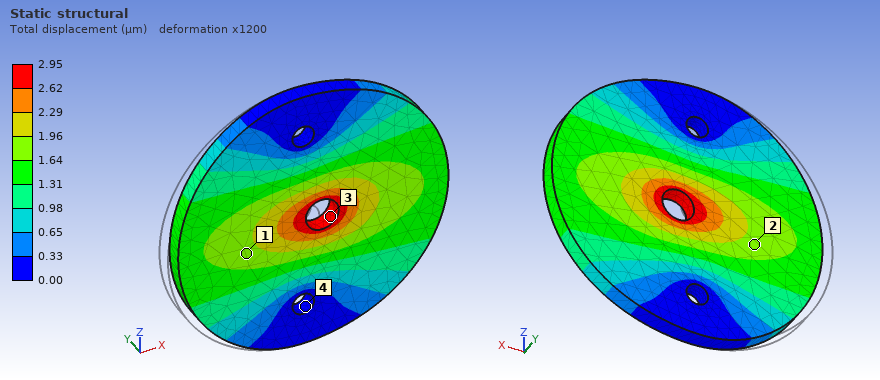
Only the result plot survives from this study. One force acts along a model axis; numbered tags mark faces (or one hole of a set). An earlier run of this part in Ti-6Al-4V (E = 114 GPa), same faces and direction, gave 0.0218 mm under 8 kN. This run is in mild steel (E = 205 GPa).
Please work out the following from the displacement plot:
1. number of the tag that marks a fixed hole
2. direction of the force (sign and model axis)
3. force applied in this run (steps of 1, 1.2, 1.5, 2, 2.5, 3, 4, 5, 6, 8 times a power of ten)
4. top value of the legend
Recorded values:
4
+X
2 kN
2.95 µm
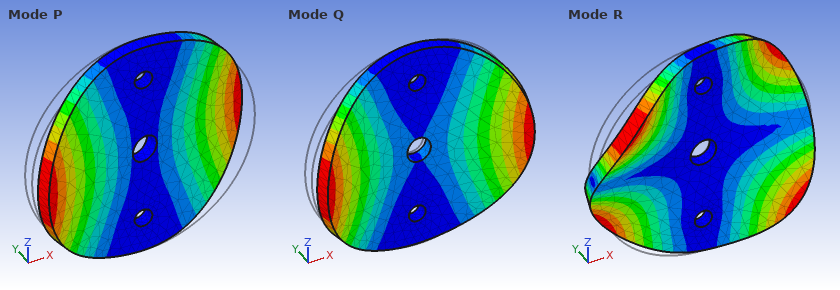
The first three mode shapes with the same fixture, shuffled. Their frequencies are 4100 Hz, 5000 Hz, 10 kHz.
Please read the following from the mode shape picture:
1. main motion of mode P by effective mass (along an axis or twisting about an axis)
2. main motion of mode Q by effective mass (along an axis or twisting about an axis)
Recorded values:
twisting about Z
along Y
